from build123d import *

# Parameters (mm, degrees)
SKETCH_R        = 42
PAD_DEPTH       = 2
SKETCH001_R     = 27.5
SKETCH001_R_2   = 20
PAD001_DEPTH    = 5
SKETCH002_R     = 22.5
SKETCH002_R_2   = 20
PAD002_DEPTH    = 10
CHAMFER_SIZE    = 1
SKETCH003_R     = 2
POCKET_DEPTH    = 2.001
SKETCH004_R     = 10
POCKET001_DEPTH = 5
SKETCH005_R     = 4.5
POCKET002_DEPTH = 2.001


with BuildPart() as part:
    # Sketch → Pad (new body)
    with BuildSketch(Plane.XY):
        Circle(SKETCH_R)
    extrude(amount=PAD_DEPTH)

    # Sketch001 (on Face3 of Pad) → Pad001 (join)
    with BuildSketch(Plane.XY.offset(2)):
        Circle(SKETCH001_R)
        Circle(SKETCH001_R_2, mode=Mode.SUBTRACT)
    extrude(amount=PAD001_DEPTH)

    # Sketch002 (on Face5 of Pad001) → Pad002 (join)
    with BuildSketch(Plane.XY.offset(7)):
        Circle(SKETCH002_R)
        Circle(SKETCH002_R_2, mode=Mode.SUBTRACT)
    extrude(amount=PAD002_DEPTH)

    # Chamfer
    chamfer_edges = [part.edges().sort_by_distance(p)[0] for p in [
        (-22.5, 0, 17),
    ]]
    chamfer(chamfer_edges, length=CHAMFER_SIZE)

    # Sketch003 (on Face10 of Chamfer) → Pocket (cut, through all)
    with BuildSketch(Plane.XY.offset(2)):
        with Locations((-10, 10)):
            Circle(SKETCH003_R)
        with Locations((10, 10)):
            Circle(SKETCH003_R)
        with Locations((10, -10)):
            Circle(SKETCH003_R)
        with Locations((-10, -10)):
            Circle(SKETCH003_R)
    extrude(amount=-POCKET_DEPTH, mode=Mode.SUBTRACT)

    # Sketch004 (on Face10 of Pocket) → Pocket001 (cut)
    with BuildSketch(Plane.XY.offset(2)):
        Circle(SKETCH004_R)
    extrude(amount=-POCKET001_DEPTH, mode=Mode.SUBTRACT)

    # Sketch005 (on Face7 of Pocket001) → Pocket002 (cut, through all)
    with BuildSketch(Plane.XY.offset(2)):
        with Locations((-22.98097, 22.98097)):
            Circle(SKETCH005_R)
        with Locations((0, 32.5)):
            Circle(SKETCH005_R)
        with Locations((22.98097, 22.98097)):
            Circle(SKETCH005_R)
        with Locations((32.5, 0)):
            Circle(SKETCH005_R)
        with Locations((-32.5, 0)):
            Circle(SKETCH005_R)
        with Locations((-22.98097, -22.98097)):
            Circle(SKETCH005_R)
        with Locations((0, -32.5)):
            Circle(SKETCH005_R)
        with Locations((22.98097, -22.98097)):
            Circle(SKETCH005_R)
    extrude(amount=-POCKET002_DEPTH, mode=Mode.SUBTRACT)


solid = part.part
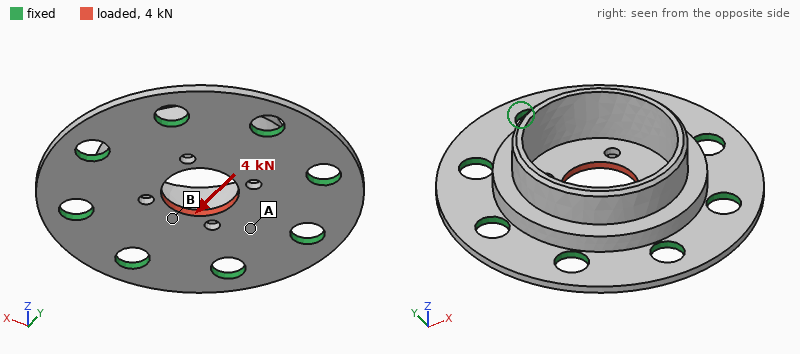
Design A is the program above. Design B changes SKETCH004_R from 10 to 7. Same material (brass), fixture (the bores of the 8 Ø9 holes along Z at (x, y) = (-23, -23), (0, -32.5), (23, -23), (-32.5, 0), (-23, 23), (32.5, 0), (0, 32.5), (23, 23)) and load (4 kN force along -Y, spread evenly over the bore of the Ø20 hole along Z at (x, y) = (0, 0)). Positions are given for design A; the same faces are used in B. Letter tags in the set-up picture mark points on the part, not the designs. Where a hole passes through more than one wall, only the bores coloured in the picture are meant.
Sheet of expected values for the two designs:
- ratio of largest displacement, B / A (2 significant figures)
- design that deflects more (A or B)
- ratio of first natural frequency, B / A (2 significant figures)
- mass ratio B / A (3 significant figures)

1.2
B
0.80
1.02
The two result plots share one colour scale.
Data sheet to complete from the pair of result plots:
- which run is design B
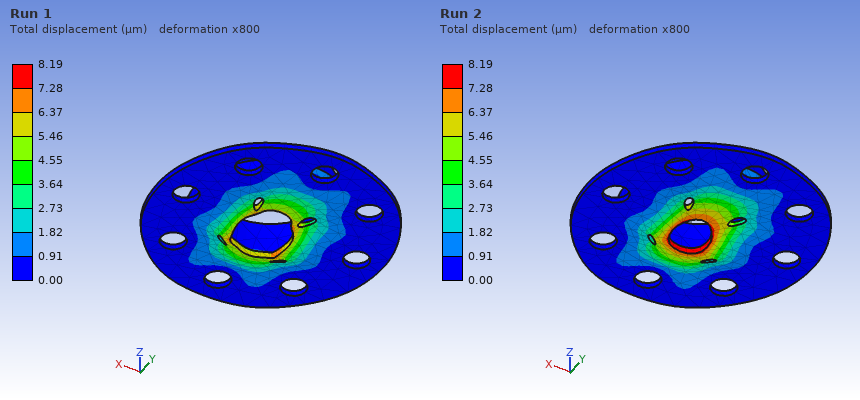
Run 2
